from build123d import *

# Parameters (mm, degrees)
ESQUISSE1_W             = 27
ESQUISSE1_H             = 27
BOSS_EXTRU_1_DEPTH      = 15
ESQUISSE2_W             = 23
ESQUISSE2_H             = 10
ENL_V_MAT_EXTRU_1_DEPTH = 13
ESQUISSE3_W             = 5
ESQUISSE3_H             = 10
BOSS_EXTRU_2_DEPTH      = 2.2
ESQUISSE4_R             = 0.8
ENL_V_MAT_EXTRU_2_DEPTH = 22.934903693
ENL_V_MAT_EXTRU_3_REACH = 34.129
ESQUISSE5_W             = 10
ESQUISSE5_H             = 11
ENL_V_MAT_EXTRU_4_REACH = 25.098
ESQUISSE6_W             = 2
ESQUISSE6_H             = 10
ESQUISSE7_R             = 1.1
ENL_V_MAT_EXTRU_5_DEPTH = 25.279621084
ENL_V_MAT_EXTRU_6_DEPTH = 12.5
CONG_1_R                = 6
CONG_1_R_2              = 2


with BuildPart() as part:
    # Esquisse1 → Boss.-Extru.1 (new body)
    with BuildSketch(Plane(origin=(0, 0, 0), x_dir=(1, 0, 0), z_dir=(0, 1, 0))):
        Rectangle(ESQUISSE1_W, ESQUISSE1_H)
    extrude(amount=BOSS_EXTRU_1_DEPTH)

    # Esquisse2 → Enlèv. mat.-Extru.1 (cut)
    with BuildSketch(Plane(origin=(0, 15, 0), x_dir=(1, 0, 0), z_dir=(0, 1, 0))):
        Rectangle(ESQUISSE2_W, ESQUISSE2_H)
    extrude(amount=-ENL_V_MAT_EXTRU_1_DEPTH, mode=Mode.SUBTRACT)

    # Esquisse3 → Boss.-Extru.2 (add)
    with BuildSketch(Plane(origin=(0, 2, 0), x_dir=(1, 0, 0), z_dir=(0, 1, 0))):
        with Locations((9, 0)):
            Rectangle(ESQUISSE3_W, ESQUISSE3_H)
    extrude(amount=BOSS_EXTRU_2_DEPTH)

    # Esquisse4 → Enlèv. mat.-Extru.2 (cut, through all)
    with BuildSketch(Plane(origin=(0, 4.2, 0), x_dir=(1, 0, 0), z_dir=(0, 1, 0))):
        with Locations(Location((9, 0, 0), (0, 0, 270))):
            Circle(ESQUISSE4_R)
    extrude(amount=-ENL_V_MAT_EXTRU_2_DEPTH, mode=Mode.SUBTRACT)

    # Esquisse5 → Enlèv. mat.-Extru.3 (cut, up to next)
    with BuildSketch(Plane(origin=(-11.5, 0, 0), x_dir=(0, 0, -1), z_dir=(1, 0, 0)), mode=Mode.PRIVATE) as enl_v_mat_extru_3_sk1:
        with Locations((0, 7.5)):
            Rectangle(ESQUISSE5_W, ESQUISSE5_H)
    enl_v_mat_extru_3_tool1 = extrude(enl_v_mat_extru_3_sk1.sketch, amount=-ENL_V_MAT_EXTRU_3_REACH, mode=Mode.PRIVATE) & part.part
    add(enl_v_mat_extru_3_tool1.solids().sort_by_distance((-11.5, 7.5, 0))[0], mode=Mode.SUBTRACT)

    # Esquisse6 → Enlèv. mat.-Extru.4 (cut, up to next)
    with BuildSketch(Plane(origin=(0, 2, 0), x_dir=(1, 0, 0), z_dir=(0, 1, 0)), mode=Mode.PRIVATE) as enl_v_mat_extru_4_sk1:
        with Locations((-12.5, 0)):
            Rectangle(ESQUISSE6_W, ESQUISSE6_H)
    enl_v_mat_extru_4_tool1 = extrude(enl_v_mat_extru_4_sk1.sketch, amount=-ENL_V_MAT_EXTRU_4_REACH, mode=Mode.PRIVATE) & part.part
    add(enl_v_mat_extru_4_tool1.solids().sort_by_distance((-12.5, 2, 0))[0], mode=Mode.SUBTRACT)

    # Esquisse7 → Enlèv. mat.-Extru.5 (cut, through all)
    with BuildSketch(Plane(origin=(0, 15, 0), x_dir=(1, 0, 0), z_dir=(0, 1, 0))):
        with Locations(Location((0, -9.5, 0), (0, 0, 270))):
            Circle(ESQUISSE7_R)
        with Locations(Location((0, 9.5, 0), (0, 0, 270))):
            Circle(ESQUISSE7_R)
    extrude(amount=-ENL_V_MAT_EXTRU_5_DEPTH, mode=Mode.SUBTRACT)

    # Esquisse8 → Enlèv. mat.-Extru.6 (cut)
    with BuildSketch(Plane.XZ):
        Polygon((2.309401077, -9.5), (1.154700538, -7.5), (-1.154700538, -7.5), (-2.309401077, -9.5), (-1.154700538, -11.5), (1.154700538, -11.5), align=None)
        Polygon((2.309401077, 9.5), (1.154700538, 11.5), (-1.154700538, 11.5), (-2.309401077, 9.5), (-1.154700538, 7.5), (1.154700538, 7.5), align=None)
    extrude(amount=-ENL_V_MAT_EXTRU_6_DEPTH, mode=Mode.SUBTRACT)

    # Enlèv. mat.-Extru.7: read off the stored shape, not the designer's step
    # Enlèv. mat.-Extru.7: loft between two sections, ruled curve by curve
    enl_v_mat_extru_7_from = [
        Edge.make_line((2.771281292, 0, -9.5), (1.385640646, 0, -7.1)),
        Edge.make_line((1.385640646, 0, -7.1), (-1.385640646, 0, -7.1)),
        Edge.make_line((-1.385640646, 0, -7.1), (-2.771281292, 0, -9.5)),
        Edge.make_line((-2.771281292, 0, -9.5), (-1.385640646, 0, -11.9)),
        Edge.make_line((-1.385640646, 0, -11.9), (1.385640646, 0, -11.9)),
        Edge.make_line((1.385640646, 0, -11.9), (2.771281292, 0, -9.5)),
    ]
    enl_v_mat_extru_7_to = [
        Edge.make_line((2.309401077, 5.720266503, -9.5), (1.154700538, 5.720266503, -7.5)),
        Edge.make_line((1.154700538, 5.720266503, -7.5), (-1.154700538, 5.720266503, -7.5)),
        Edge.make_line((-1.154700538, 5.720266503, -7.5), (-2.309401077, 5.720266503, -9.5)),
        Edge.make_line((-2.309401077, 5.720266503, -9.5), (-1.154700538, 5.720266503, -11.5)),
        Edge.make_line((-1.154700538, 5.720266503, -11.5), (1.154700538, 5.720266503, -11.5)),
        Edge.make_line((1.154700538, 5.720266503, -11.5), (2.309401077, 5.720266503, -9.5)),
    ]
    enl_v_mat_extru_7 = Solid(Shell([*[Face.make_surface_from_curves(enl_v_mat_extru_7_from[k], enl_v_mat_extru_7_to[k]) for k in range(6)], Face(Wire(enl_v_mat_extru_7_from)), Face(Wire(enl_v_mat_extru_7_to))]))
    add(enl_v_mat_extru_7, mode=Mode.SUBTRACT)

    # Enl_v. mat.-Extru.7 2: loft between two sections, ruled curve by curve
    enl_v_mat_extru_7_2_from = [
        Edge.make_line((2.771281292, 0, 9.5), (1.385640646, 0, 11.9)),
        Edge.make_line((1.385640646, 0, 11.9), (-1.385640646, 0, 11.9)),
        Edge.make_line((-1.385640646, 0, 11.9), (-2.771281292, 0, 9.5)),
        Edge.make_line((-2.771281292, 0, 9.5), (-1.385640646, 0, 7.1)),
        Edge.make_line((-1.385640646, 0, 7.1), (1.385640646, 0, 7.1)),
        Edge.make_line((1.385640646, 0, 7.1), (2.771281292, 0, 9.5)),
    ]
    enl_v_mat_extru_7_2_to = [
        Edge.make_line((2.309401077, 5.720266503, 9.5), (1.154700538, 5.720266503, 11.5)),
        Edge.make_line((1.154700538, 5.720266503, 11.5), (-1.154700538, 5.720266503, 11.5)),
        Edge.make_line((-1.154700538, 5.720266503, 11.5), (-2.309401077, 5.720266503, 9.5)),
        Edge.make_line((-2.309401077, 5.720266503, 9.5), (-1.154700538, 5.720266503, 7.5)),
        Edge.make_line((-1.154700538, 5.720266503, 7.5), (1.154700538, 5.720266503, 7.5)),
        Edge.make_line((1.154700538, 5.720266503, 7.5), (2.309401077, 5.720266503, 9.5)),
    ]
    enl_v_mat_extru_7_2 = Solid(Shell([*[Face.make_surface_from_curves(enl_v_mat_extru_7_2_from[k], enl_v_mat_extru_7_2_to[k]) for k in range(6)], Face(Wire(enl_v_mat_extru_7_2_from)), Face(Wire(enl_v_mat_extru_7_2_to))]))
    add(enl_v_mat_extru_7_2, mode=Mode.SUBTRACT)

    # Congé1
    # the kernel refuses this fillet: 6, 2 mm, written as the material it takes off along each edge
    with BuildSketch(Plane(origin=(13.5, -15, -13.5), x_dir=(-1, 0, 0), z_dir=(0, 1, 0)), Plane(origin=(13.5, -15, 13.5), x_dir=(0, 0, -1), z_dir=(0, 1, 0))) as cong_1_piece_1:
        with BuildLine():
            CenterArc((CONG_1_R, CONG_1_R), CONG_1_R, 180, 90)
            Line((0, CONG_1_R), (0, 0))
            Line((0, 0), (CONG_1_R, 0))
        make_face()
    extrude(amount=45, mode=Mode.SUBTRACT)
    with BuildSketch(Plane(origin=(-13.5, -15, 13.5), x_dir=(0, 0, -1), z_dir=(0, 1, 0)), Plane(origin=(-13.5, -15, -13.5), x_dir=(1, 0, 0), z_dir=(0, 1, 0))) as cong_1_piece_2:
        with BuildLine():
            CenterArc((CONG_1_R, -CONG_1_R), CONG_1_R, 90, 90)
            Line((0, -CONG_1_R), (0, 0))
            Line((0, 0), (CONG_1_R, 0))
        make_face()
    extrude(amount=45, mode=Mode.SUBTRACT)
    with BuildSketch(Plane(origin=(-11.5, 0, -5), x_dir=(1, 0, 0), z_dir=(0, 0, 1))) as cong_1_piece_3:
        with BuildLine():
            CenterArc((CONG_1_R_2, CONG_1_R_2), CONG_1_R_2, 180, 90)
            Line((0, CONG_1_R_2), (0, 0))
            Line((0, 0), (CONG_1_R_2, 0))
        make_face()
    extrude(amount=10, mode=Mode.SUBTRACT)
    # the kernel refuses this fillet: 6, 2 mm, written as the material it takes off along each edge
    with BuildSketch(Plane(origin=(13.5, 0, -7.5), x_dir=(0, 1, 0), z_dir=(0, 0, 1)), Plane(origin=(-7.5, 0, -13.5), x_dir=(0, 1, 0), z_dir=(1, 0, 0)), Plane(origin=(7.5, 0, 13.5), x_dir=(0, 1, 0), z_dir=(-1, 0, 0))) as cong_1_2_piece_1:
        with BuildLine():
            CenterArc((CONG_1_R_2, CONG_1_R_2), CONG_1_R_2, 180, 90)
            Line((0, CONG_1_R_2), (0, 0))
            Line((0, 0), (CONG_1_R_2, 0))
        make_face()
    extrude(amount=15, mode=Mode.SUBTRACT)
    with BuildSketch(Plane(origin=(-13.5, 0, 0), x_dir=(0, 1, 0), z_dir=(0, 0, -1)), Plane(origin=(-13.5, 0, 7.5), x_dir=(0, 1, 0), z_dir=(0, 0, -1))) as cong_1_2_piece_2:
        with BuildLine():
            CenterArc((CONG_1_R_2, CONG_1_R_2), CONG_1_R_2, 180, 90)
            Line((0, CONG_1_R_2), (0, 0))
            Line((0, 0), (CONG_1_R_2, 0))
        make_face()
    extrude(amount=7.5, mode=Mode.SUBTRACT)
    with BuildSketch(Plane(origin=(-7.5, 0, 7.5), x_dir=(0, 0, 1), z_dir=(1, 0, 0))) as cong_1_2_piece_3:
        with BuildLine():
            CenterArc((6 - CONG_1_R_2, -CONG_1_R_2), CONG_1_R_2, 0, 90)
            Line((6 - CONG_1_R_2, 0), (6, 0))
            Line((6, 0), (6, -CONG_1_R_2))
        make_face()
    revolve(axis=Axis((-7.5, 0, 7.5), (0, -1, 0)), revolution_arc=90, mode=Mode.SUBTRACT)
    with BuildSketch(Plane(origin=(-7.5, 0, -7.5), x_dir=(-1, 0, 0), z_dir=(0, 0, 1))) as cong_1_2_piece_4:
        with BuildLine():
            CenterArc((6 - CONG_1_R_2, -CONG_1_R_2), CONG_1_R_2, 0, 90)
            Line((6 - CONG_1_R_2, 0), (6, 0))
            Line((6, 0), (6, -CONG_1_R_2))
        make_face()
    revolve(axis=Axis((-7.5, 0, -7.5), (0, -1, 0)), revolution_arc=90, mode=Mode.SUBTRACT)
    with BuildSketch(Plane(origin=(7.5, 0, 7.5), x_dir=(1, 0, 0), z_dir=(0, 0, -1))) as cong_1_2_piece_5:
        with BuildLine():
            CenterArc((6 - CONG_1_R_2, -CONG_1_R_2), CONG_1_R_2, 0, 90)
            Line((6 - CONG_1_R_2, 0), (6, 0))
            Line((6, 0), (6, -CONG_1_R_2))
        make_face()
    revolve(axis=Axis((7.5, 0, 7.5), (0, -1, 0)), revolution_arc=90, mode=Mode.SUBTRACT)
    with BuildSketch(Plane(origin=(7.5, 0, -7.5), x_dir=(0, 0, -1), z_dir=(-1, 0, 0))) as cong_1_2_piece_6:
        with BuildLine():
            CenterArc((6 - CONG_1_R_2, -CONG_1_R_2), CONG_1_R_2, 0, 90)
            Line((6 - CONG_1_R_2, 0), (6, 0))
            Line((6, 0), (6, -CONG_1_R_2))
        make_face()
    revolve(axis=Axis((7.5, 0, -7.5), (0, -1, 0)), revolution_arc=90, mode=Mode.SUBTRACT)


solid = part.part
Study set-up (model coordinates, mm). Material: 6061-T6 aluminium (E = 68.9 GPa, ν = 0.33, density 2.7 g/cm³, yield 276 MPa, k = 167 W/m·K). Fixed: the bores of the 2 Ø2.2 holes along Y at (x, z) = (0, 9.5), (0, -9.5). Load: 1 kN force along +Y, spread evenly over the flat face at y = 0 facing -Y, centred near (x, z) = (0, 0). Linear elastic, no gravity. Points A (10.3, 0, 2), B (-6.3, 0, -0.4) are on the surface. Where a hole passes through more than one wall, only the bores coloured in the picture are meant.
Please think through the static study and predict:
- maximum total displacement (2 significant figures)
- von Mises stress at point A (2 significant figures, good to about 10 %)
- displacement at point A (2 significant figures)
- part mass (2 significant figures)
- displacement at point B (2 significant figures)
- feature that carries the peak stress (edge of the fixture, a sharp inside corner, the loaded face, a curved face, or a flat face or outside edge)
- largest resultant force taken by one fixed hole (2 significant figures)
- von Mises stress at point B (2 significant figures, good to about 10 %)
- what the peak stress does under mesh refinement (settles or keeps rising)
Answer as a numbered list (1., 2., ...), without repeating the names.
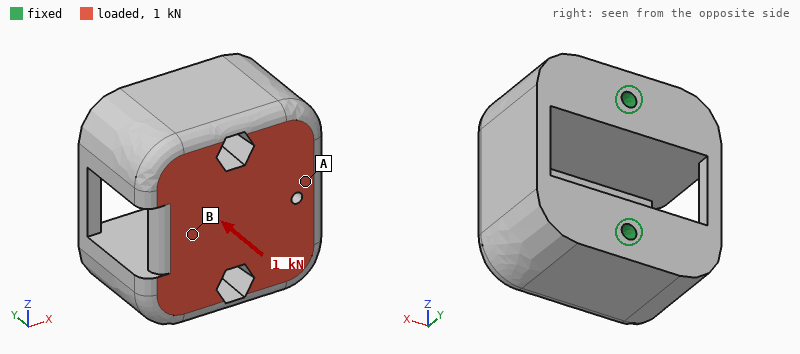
1. 7.3 µm
2. 6.6 MPa
3. 7.0 µm
4. 18 g
5. 5.4 µm
6. edge of the fixture
7. 510 N
8. 17 MPa
9. keeps rising
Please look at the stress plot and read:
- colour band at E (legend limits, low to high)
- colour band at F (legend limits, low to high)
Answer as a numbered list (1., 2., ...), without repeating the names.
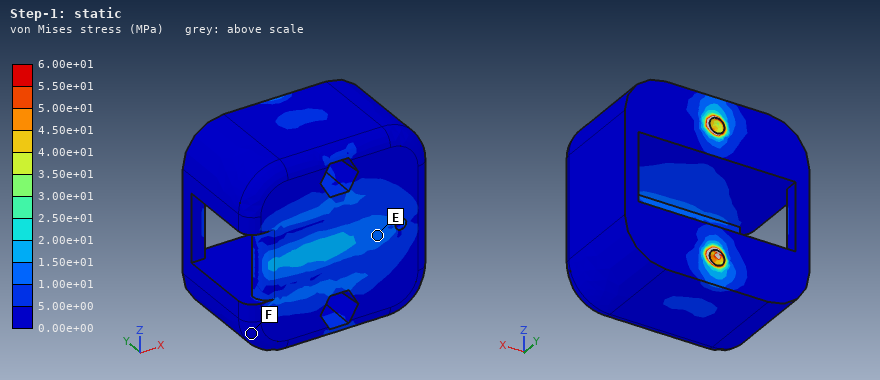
1. 1.00e+01 to 1.50e+01 MPa
2. 0.00e+00 to 5.00e+00 MPa
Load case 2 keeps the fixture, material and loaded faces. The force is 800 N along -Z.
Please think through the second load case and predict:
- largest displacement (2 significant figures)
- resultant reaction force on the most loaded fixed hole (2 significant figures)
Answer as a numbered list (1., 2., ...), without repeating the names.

1. 32 µm
2. 600 N
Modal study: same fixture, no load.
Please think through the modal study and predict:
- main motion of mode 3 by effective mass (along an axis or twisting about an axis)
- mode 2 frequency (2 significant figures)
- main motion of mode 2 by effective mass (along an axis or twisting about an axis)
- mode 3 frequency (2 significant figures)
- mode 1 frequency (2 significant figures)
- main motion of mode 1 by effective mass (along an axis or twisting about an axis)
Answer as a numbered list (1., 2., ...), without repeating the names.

1. along Z
2. 8600 Hz
3. along Z
4. 13 kHz
5. 4300 Hz
6. along X
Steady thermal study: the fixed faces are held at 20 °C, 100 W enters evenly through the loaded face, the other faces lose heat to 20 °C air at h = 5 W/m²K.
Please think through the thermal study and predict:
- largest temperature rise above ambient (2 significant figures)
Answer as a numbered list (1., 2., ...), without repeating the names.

1. 59 K
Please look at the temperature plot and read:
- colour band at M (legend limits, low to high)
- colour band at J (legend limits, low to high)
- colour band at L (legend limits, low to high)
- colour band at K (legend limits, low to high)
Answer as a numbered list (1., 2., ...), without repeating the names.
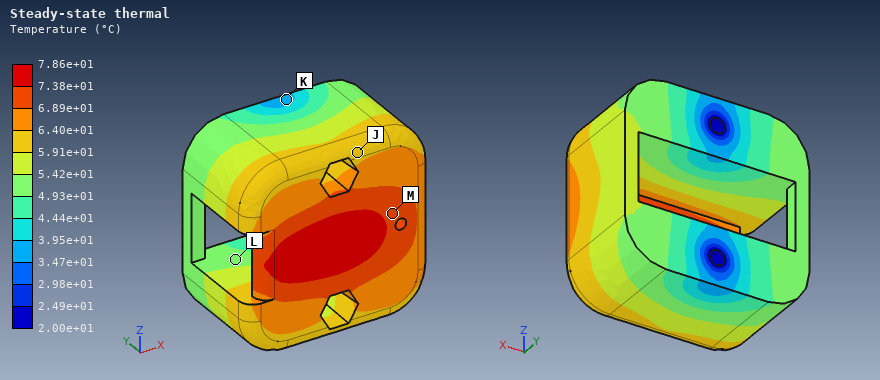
1. 6.89e+01 to 7.38e+01 °C
2. 5.91e+01 to 6.40e+01 °C
3. 4.93e+01 to 5.42e+01 °C
4. 3.47e+01 to 3.95e+01 °C
